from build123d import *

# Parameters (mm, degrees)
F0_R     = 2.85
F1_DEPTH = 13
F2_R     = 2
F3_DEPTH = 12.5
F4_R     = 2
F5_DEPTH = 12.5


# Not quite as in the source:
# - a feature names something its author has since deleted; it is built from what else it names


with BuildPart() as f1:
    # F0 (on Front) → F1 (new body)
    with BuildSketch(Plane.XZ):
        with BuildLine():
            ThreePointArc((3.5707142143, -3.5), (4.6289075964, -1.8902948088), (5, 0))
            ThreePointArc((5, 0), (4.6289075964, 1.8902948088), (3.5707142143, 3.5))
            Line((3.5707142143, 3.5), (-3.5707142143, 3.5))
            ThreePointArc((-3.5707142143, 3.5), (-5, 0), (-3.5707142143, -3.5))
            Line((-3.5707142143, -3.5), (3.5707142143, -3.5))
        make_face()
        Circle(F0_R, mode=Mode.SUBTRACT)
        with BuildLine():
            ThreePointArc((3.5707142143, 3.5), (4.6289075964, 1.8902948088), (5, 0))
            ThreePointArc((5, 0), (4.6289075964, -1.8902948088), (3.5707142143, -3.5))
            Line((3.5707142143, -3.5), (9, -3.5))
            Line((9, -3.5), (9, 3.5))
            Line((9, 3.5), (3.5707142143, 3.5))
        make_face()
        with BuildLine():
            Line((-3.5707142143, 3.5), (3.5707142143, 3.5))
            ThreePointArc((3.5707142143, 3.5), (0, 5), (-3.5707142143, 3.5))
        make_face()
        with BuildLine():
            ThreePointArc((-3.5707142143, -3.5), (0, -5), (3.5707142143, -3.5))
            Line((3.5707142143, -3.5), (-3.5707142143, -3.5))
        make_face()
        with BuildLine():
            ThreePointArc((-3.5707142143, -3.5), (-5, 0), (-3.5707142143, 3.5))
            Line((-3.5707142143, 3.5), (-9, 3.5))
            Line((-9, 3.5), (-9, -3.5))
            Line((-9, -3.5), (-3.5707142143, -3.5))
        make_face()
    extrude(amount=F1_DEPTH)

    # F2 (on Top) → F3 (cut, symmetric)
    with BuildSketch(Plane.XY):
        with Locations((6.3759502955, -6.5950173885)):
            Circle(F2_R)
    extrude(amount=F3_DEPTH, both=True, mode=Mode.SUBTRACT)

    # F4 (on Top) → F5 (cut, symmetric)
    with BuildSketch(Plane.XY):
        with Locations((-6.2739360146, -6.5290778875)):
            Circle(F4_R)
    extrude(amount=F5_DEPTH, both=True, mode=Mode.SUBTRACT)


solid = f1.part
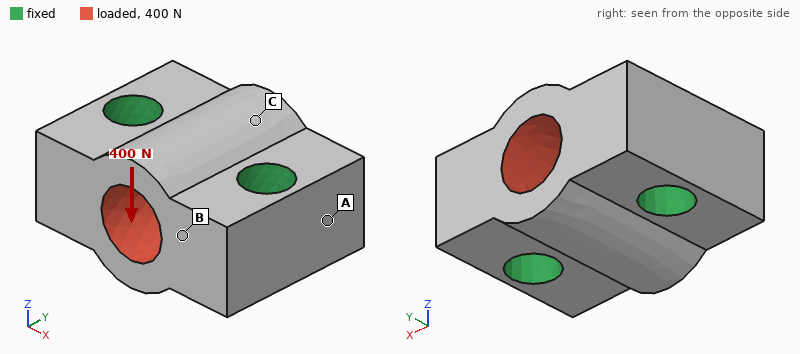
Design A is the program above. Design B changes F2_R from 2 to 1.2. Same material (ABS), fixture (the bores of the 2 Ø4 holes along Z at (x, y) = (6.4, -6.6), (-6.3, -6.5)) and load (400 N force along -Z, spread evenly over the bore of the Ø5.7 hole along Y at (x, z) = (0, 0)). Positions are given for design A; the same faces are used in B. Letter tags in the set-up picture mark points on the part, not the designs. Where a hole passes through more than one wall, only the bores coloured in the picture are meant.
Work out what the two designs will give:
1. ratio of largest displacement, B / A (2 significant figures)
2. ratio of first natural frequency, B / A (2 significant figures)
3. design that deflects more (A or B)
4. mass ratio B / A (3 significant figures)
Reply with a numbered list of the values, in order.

1. 1.1
2. 0.86
3. B
4. 1.04
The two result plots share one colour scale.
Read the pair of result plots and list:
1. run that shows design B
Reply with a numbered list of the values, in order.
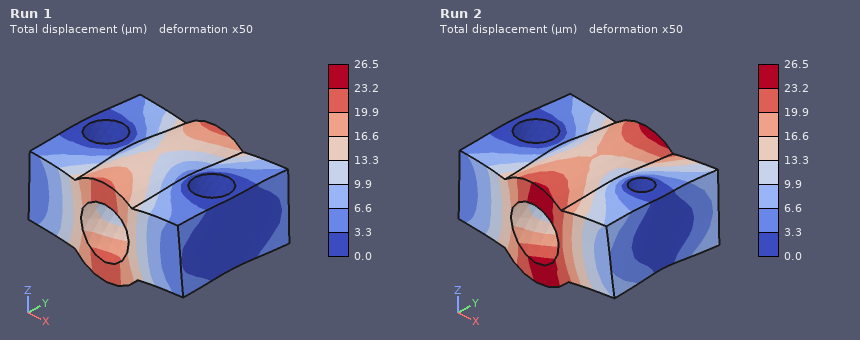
1. Run 2
